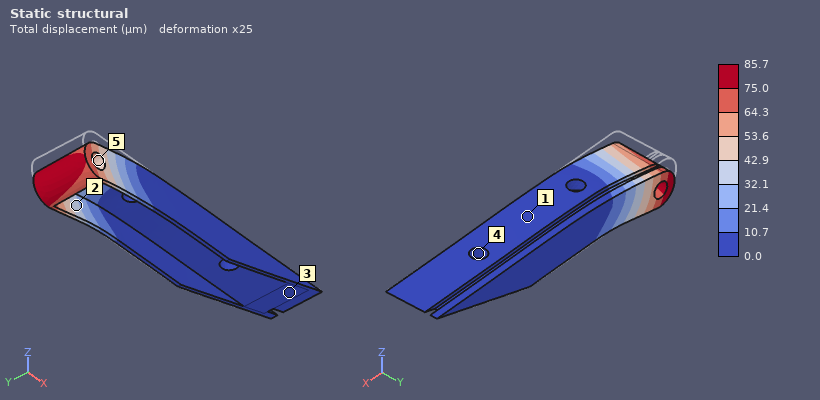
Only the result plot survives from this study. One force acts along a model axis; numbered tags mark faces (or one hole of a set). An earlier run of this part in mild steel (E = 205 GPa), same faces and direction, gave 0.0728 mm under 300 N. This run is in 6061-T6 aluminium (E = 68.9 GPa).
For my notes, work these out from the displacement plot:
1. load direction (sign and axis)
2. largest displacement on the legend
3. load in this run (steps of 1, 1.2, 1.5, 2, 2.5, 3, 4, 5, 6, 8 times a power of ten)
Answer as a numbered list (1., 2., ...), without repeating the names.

1. -Z
2. 85.7 µm
3. 120 N
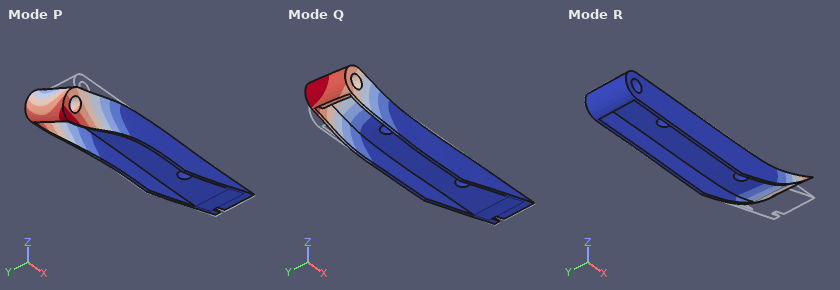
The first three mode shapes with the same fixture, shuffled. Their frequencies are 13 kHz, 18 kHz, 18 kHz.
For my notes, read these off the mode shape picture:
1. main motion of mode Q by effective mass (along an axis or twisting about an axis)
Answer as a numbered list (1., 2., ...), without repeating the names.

1. along Z
